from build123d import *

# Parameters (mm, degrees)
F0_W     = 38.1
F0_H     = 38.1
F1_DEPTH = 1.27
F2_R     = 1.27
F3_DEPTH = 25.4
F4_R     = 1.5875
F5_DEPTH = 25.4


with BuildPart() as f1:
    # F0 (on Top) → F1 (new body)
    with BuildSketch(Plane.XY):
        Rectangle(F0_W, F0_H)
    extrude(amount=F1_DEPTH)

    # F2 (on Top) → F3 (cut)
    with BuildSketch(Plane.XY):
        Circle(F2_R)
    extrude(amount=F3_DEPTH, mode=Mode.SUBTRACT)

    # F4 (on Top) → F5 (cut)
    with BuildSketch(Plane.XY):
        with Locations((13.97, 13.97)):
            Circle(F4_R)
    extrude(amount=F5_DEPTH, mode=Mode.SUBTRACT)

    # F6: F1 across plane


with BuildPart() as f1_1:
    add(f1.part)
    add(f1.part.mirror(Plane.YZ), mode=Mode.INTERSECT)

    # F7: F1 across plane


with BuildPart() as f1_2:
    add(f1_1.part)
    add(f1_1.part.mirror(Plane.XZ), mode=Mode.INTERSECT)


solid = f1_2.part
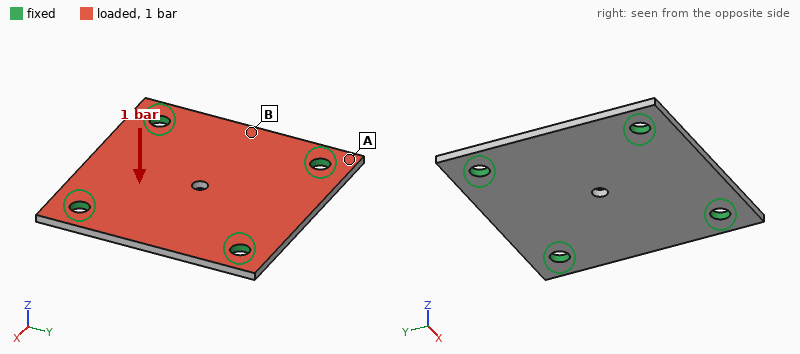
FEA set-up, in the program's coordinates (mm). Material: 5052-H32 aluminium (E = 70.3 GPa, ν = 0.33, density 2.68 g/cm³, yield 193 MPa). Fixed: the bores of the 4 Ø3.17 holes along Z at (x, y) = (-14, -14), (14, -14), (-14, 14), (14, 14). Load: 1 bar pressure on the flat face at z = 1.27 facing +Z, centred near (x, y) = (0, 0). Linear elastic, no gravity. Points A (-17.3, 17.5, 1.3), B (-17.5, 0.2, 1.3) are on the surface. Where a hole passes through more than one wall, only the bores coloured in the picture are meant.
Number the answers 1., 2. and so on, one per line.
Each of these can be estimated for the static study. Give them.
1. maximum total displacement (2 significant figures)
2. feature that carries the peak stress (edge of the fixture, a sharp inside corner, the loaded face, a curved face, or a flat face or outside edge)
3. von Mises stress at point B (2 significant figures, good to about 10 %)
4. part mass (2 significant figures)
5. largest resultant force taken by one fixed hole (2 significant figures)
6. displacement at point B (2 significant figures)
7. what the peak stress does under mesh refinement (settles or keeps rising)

1. 26 µm
2. edge of the fixture
3. 12 MPa
4. 4.8 g
5. 35 N
6. 11 µm
7. keeps rising
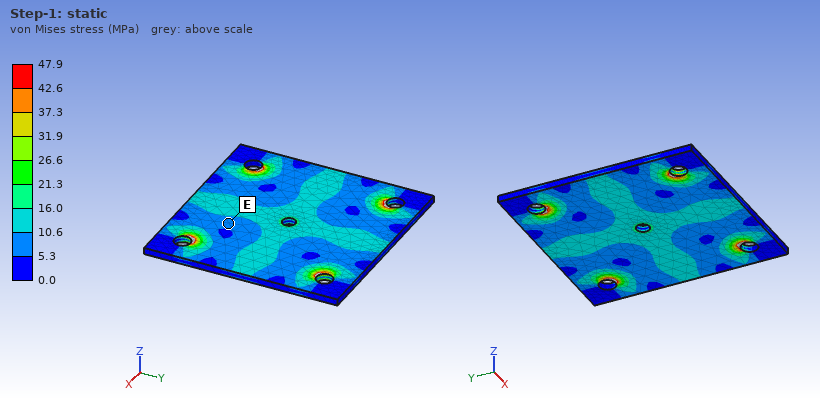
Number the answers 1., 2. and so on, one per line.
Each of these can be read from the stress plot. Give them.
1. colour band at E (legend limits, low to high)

1. 5.3 to 10.6 MPa
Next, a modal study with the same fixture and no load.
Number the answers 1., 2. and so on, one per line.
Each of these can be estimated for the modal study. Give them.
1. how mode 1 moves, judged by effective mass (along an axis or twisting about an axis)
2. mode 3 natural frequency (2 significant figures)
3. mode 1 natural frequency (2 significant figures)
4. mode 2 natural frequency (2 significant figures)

1. along Z
2. 10 kHz
3. 6700 Hz
4. 10 kHz
